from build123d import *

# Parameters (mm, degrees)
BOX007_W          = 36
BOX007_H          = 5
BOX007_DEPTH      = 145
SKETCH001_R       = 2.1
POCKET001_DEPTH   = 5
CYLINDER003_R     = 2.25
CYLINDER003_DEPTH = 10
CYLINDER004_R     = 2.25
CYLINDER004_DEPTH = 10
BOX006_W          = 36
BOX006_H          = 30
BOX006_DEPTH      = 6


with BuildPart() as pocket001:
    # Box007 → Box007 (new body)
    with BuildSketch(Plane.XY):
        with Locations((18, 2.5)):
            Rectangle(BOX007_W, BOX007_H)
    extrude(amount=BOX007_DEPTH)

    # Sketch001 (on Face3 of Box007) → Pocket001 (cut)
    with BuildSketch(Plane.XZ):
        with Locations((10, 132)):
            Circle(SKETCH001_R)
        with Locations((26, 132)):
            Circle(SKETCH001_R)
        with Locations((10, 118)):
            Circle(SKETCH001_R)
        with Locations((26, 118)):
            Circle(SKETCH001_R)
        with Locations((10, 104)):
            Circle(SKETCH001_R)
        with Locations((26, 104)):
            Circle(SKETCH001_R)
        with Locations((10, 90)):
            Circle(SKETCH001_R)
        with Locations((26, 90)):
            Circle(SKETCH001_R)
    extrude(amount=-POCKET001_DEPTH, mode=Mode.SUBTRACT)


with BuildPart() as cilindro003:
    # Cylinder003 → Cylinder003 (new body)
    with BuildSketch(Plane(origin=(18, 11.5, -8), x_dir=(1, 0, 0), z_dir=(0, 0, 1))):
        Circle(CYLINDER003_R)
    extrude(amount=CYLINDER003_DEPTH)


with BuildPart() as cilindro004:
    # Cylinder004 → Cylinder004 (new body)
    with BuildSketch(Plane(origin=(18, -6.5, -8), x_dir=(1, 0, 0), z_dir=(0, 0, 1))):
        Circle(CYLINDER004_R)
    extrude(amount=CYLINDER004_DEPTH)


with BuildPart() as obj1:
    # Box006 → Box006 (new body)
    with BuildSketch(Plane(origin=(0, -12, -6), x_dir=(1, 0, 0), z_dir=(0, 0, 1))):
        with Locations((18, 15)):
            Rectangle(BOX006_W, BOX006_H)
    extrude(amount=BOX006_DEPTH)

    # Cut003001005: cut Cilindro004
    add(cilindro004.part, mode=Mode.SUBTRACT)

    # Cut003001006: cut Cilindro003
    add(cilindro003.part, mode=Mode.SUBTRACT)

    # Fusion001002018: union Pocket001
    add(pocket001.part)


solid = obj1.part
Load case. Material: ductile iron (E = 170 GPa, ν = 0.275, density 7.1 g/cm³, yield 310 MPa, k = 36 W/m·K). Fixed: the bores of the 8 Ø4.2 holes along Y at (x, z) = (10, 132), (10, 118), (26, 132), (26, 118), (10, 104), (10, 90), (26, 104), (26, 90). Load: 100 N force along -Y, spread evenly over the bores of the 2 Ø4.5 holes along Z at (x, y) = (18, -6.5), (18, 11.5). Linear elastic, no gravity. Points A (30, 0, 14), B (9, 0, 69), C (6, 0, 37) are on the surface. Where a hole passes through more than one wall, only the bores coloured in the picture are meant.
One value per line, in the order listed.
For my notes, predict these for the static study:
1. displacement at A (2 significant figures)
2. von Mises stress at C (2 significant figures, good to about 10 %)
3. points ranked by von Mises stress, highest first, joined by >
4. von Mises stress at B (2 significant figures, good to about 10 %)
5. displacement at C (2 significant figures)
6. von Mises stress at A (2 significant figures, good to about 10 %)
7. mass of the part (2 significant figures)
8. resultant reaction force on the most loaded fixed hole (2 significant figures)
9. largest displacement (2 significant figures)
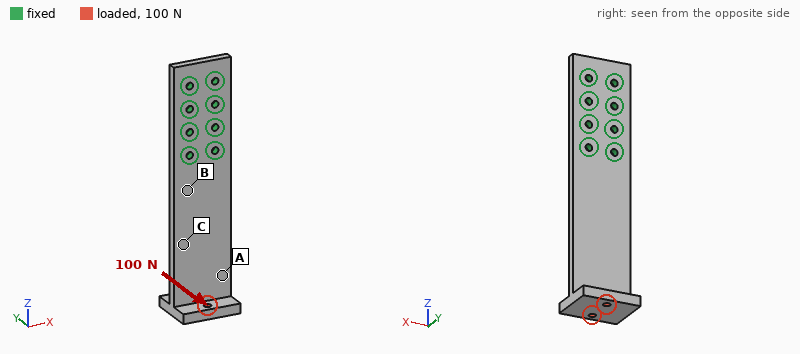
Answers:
0.30 mm
27 MPa
B > C > A
46 MPa
0.16 mm
12 MPa
230 g
140 N
0.44 mm
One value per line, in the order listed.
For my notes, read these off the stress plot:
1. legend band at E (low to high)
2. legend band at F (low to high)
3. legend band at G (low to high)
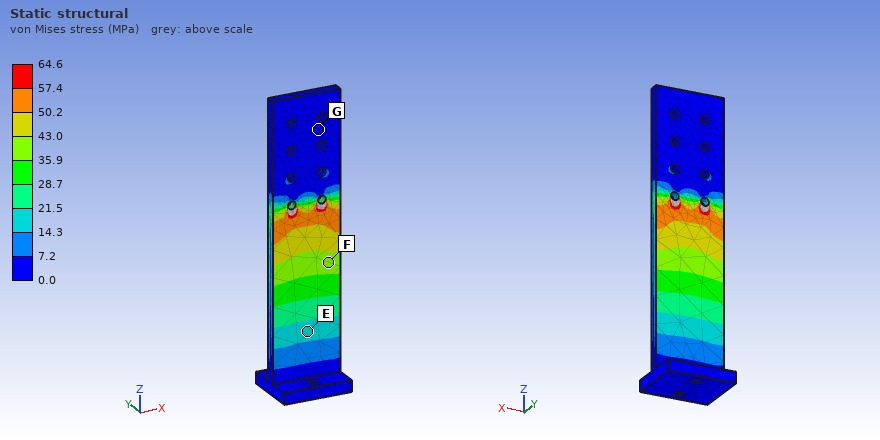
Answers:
14.3 to 21.5 MPa
35.9 to 43.0 MPa
0.0 to 7.2 MPa
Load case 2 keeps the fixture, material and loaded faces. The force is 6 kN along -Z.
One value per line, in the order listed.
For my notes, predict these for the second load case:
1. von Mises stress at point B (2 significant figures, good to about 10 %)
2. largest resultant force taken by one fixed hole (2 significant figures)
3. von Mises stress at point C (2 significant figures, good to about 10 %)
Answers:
34 MPa
2.5 kN
33 MPa
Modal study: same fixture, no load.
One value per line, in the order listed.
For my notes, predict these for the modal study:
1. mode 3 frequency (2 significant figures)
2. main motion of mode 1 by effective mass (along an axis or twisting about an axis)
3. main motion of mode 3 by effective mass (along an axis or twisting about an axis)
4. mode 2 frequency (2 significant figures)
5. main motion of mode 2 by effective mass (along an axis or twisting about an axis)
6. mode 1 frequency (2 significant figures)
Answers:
1800 Hz
along Y
along X
1500 Hz
twisting about Z
300 Hz
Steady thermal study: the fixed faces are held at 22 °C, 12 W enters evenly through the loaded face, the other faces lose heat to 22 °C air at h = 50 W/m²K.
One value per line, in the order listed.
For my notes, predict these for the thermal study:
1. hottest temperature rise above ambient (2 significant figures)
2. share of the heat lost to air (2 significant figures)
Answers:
50 K
89 %
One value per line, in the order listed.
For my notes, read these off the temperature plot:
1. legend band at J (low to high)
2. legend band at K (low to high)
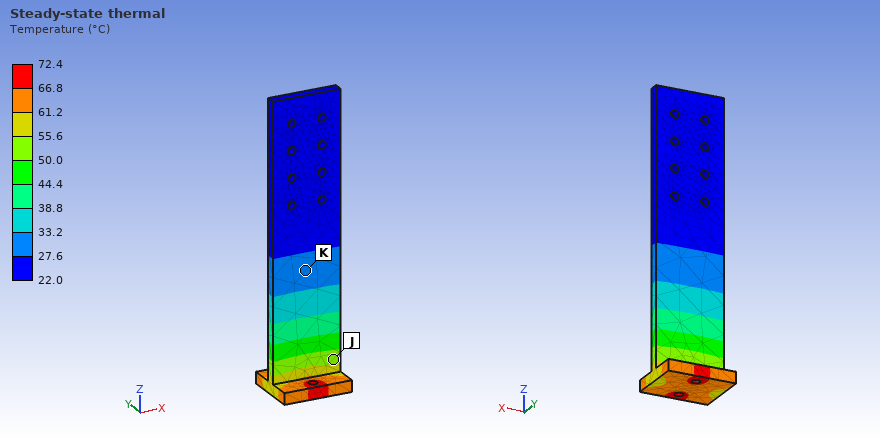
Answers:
50.0 to 55.6 °C
27.6 to 33.2 °C
